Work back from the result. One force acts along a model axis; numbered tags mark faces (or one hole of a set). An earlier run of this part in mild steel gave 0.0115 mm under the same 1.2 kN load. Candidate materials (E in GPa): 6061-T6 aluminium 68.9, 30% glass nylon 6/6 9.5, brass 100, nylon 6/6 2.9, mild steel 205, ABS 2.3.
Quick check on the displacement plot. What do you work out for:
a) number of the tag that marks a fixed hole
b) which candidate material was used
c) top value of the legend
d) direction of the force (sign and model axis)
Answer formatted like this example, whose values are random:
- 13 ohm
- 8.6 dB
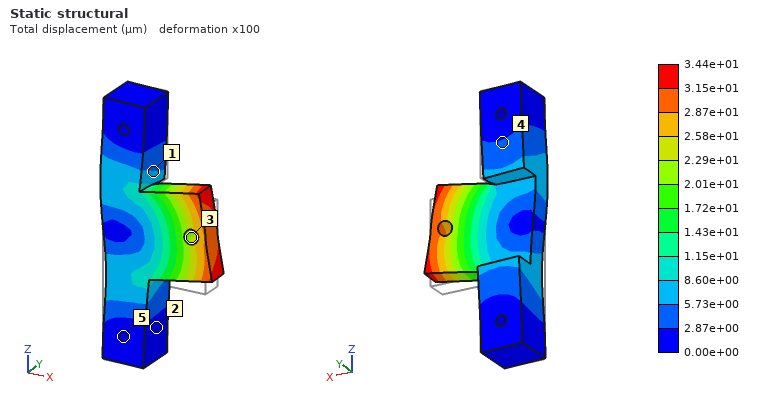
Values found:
- 5
- 6061-T6 aluminium
- 3.44e+01 µm
- +Z
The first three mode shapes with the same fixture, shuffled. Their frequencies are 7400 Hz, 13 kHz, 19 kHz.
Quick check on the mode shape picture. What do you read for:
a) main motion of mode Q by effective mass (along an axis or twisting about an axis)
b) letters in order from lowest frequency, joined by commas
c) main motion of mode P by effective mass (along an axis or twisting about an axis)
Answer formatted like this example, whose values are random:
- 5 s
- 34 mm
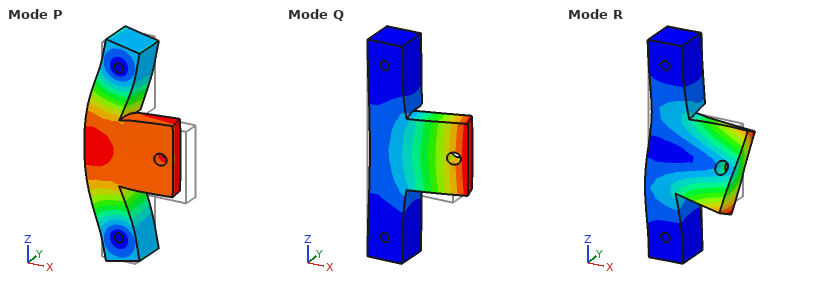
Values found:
- along Y
- Q, P, R
- along X
